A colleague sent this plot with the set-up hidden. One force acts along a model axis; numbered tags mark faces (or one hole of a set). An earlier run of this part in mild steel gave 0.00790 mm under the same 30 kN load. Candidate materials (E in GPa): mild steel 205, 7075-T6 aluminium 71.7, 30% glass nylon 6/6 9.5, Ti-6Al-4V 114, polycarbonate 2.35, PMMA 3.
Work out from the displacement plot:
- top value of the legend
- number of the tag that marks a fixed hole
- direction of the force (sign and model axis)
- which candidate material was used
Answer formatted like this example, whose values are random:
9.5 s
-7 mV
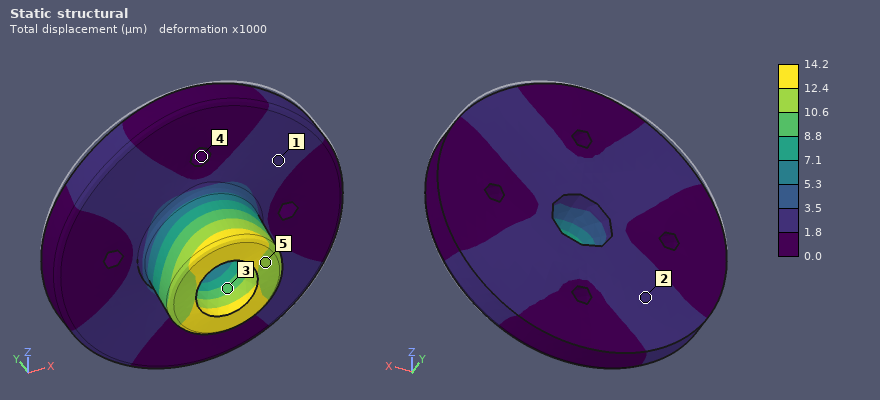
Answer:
14.2 µm
4
-Z
Ti-6Al-4V
